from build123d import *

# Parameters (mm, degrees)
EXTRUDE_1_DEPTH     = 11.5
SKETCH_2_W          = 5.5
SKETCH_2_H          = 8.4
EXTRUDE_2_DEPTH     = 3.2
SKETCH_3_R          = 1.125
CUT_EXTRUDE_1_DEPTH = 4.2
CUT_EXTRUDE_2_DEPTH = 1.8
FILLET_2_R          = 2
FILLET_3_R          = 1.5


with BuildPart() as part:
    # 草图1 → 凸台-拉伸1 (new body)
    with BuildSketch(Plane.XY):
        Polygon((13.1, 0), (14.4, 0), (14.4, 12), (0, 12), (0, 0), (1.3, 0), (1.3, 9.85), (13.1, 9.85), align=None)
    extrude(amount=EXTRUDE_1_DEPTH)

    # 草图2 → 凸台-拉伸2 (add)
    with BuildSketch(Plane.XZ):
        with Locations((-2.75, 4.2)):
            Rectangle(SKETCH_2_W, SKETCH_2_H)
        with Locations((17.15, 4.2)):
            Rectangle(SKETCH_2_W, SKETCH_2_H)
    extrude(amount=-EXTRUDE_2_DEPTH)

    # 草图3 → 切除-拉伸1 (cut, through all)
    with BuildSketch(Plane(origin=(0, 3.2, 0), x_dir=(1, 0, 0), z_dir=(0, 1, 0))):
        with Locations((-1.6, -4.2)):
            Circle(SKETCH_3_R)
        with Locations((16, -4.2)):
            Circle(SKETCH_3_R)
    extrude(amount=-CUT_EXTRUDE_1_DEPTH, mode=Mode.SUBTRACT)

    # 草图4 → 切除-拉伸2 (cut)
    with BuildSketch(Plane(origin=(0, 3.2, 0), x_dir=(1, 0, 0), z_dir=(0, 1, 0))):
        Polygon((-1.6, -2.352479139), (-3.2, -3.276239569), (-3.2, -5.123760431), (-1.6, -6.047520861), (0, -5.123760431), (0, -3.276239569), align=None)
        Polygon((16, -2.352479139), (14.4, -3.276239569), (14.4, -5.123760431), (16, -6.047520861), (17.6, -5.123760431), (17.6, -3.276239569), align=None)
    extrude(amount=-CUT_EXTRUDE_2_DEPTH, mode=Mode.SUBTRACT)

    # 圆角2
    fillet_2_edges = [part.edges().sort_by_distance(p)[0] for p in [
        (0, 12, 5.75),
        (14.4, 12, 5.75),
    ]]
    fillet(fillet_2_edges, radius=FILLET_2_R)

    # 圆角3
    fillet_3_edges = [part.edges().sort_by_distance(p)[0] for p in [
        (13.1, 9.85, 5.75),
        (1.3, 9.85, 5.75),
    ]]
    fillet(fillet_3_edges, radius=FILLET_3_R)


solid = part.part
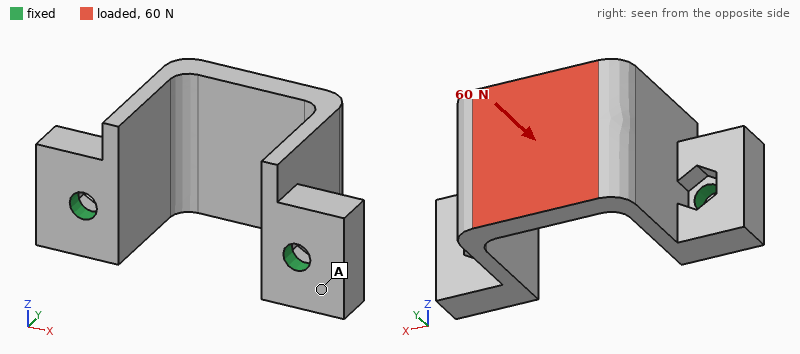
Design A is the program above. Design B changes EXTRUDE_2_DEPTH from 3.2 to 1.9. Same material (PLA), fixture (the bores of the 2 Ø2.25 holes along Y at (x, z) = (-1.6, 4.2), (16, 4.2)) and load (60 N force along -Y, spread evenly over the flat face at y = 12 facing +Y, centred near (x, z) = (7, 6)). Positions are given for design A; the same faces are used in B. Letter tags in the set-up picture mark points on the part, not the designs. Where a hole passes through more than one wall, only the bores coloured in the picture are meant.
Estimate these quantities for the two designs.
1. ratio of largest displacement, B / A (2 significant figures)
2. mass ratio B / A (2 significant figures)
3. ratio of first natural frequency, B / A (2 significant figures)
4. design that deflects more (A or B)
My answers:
1.3
0.89
0.85
B
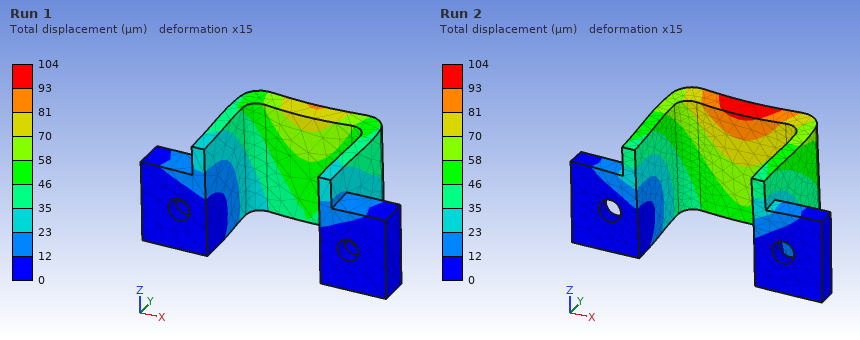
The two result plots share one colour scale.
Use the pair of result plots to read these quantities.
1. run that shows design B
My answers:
Run 2
